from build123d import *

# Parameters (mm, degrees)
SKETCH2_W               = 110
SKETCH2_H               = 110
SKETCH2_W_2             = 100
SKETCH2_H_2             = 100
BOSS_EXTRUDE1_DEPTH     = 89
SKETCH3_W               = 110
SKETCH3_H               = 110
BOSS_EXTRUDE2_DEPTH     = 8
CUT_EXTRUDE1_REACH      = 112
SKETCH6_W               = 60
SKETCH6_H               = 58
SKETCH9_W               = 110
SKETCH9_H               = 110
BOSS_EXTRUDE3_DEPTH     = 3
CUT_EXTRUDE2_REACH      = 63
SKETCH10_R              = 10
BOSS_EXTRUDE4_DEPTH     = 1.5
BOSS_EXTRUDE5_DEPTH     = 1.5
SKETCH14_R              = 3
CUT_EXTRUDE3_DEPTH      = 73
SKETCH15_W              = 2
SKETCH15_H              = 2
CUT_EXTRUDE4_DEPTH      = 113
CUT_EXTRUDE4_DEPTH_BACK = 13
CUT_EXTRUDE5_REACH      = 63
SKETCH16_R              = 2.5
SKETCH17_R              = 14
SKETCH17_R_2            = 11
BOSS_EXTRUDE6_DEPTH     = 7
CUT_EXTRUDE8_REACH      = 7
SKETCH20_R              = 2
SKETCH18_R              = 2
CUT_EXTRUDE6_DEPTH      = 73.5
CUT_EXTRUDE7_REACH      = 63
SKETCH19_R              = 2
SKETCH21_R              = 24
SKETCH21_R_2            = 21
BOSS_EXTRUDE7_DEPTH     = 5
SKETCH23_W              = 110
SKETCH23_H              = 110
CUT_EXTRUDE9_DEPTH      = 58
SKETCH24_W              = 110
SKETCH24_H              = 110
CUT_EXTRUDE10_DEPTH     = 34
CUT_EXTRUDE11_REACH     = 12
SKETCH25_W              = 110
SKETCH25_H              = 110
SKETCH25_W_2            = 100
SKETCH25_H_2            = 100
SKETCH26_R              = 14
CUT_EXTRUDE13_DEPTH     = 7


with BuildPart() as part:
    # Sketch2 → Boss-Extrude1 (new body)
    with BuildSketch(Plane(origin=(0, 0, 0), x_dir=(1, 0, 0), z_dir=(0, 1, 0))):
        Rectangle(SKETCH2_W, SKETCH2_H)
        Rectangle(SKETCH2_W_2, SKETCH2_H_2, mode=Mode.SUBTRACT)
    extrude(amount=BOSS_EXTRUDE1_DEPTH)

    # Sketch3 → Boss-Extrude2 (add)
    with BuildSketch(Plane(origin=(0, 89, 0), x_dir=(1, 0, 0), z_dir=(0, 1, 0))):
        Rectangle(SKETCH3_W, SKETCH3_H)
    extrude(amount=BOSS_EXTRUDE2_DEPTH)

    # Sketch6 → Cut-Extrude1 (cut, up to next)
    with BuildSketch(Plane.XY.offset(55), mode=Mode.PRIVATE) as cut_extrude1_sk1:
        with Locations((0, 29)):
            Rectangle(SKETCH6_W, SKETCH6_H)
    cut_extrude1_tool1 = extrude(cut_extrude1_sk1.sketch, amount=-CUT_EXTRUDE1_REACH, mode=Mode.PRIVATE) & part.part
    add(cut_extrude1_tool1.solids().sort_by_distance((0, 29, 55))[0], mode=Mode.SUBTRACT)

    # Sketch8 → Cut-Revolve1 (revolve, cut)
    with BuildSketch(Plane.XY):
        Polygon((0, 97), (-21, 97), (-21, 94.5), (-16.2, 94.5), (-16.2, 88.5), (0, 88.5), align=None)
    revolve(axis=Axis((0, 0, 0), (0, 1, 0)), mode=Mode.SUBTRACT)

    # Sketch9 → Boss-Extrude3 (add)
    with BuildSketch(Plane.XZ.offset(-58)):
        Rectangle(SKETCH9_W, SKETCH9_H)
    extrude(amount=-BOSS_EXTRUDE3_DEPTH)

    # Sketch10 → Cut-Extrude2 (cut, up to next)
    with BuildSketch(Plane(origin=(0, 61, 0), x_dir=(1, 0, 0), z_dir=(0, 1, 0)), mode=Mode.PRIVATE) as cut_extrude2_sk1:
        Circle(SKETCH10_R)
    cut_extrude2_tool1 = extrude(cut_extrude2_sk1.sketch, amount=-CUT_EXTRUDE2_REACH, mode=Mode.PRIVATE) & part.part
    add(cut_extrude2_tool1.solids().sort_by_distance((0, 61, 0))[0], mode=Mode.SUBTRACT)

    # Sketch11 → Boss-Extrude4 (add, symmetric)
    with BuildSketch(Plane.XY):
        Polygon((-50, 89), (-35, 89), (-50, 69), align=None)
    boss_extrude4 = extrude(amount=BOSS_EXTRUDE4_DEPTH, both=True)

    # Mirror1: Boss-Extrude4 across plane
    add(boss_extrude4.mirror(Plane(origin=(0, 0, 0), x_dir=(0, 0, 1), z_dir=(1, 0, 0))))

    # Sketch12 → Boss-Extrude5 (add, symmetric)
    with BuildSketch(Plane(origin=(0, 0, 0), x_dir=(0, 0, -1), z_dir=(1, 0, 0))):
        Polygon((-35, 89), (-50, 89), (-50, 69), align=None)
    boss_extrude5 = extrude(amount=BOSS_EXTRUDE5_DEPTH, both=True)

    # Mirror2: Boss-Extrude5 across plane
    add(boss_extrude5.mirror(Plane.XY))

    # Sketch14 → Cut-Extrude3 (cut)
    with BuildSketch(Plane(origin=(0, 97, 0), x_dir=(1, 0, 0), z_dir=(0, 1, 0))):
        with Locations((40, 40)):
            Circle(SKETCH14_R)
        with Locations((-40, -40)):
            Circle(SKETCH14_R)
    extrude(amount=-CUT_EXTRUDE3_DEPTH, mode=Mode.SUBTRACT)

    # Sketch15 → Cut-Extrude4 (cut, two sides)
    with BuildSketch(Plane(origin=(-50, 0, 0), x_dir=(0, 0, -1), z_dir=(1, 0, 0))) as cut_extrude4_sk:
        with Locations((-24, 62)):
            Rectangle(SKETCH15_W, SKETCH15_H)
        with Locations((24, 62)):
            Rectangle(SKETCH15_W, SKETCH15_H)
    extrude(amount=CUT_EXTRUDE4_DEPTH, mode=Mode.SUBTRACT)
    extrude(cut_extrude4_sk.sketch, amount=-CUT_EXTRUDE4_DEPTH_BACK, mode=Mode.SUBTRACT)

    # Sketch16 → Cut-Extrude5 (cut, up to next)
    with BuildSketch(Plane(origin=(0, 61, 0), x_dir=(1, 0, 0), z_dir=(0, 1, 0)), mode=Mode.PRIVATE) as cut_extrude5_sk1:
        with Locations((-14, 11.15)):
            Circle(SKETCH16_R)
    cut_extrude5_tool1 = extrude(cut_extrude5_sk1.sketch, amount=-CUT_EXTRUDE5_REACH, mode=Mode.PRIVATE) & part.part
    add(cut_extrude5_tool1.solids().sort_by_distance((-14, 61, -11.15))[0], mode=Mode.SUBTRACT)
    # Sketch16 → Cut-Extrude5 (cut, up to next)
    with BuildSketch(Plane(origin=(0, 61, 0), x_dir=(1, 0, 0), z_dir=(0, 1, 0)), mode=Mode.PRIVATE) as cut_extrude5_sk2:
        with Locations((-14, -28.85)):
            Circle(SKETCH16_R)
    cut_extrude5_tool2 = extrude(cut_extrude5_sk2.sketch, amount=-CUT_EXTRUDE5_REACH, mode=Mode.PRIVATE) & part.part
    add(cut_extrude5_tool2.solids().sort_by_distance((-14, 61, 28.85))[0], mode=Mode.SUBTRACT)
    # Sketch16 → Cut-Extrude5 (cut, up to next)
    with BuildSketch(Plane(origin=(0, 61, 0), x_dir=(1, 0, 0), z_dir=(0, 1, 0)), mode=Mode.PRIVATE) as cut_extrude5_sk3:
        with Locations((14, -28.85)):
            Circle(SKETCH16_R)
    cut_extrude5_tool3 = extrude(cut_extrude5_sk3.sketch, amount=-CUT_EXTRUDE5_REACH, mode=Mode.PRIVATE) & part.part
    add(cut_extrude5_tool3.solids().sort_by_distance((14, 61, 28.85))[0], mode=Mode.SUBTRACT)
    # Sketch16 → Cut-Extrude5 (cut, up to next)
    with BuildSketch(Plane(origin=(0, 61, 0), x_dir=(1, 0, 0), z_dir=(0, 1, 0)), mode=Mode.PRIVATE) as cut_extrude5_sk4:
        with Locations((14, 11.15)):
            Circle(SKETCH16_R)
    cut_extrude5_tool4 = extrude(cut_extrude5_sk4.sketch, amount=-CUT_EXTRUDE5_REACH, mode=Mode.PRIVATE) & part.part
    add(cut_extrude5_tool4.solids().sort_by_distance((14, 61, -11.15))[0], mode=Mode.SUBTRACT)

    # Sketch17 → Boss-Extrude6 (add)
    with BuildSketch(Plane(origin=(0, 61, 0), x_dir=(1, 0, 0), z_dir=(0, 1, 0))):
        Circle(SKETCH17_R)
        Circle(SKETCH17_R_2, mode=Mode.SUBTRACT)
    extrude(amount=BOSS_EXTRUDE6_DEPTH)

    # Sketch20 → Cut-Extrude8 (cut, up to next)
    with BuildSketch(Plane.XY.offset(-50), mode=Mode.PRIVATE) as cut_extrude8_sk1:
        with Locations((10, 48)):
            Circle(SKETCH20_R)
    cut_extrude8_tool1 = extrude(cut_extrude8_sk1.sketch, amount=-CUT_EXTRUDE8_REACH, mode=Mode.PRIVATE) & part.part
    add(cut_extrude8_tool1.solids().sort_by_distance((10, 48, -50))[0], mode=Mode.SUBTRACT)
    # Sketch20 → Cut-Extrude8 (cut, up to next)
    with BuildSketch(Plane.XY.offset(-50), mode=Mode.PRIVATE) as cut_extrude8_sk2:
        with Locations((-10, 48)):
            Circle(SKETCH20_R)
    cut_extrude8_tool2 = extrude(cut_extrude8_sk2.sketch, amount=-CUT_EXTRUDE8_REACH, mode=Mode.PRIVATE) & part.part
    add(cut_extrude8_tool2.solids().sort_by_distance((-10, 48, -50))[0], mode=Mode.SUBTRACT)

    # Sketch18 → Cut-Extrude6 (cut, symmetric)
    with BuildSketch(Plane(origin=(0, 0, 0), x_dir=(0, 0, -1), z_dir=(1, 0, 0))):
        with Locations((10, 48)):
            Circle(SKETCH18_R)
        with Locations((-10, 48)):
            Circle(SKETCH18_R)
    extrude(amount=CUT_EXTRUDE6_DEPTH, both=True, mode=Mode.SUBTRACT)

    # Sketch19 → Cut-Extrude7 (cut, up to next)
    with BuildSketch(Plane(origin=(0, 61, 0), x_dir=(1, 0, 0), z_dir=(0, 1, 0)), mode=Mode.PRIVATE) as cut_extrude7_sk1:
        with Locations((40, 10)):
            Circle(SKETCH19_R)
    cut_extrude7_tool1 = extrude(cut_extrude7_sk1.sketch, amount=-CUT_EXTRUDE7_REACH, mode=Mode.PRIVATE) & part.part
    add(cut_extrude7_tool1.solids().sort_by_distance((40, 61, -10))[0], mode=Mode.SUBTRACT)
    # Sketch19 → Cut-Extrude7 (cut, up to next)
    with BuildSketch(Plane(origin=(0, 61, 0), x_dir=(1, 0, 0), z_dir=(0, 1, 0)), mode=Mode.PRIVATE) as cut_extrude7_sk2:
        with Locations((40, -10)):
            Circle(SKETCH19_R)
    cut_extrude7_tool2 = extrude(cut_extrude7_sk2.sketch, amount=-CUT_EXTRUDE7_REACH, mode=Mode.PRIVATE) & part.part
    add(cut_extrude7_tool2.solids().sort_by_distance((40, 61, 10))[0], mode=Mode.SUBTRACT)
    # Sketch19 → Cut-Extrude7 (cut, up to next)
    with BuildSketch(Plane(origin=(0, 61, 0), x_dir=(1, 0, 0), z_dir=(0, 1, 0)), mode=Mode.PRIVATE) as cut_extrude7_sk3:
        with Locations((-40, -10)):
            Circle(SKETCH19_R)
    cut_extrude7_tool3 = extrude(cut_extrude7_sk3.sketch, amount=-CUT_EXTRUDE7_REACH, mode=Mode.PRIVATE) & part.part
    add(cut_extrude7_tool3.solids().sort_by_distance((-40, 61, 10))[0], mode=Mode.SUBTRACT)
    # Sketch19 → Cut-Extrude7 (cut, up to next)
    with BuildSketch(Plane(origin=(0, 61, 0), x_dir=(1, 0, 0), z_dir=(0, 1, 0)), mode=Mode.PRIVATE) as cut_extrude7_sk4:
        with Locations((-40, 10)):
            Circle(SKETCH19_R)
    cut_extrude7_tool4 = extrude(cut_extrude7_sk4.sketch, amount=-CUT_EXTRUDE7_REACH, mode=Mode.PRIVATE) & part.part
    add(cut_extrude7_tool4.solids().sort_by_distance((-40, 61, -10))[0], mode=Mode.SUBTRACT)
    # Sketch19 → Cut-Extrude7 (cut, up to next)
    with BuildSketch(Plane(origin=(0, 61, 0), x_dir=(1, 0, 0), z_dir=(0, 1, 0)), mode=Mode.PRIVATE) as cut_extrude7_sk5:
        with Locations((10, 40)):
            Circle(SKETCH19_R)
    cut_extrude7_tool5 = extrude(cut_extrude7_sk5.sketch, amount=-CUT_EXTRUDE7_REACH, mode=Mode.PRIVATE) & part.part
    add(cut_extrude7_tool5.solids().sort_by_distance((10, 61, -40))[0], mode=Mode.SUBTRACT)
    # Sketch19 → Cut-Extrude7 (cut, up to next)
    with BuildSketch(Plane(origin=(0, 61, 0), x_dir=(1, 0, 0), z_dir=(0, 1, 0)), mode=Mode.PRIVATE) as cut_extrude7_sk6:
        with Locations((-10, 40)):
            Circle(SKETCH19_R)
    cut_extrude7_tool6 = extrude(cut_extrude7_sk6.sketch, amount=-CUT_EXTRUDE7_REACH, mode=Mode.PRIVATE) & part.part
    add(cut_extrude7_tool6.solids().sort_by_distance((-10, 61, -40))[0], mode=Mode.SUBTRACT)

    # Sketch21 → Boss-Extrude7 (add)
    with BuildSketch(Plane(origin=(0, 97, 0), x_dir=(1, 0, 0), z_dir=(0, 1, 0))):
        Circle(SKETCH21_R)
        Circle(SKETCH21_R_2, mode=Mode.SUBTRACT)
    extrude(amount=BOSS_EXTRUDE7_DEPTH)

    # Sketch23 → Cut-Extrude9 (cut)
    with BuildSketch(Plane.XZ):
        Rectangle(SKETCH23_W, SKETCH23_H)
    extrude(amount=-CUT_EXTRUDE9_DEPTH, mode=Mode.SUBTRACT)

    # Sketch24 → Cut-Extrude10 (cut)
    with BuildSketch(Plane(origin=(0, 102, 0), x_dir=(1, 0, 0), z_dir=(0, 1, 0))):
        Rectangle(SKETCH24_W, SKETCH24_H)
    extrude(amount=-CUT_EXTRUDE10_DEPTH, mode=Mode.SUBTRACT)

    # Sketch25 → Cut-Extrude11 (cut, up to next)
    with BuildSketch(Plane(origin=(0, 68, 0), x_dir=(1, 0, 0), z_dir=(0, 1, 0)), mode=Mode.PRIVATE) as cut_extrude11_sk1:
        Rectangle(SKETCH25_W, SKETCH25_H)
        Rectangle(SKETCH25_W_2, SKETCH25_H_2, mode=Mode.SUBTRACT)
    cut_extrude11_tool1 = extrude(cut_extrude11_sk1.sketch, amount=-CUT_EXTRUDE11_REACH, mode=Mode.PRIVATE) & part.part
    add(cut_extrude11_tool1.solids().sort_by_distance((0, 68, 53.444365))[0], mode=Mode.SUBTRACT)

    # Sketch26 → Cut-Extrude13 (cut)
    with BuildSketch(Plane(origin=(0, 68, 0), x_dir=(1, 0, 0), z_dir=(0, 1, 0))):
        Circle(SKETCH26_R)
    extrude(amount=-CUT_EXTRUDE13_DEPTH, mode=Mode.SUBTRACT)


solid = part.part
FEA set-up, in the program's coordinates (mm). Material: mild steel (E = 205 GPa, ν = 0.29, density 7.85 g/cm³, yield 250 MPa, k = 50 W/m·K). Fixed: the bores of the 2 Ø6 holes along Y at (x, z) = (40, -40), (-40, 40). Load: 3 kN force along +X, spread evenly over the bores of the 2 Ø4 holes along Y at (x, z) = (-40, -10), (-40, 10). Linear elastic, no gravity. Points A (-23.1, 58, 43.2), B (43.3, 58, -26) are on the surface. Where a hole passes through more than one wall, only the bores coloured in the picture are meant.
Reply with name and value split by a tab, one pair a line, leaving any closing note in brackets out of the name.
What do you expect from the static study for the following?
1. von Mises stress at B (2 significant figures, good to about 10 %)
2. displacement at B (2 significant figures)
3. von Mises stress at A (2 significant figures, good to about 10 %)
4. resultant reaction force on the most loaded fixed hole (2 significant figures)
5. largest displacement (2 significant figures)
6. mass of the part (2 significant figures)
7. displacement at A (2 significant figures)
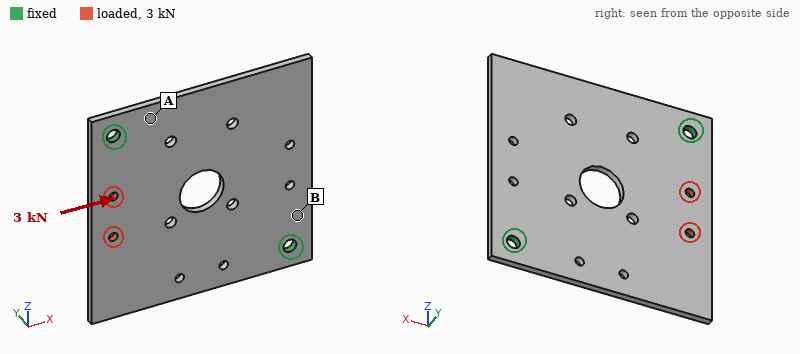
von Mises stress at B	8.1 MPa
displacement at B	2.0 µm
von Mises stress at A	19 MPa
resultant reaction force on the most loaded fixed hole	1.6 kN
largest displacement	9.9 µm
mass of the part	220 g
displacement at A	2.4 µm
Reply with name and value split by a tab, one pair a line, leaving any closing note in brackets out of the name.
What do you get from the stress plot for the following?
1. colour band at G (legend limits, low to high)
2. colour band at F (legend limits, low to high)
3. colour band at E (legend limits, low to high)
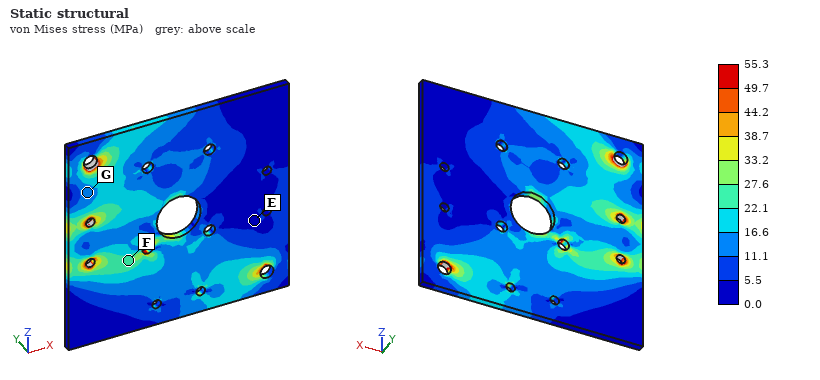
colour band at G	11.1 to 16.6 MPa
colour band at F	22.1 to 27.6 MPa
colour band at E	0.0 to 5.5 MPa
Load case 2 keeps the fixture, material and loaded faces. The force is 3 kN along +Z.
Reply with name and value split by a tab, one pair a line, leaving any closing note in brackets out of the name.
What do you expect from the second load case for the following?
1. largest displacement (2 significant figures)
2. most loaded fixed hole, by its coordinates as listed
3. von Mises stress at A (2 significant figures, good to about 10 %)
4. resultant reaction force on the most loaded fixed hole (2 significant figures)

largest displacement	8.7 µm
most loaded fixed hole, by its coordinates as listed	(-40, 40)
von Mises stress at A	12 MPa
resultant reaction force on the most loaded fixed hole	2.6 kN
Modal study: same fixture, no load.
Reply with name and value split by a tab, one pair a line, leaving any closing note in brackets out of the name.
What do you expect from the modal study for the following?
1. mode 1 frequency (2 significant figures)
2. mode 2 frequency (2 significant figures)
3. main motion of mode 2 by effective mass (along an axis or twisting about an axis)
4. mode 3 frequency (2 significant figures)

mode 1 frequency	500 Hz
mode 2 frequency	670 Hz
main motion of mode 2 by effective mass	along Y
mode 3 frequency	1700 Hz
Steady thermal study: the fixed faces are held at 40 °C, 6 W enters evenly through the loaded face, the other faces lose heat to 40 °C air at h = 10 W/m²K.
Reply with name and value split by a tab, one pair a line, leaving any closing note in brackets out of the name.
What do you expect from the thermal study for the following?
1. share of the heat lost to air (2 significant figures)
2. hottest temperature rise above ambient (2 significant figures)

share of the heat lost to air	32 %
hottest temperature rise above ambient	28 K
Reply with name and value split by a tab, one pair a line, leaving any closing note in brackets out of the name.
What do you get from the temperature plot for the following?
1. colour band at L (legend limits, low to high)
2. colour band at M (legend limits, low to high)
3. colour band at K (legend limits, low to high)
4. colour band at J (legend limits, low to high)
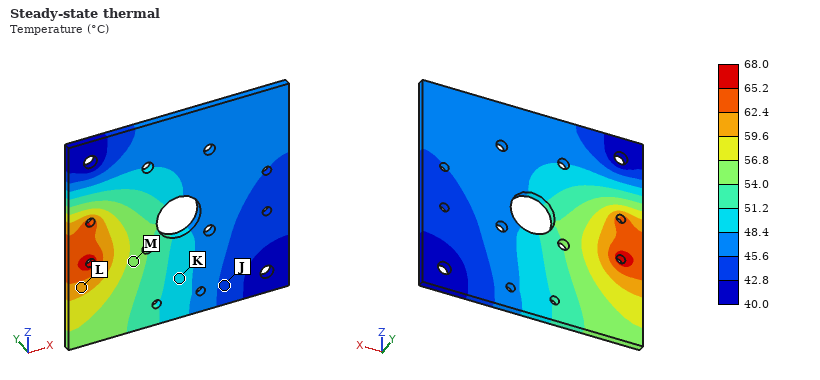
colour band at L	59.6 to 62.4 °C
colour band at M	54.0 to 56.8 °C
colour band at K	48.4 to 51.2 °C
colour band at J	42.8 to 45.6 °C
